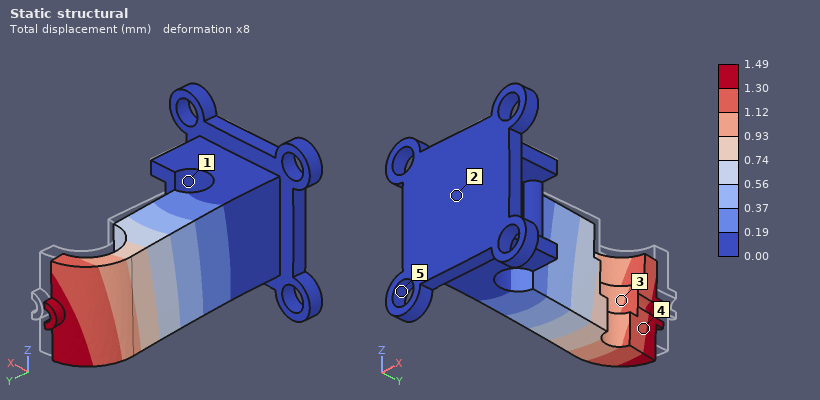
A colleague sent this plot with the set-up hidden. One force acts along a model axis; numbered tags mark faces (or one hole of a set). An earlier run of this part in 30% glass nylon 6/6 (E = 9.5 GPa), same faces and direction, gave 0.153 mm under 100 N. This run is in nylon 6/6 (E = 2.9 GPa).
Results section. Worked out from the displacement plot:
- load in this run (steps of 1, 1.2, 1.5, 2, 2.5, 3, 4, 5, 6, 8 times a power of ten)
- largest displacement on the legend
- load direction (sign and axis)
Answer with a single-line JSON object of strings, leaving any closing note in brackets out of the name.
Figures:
{"load in this run": "300 N", "largest displacement on the legend": "1.49 mm", "load direction": "-X"}
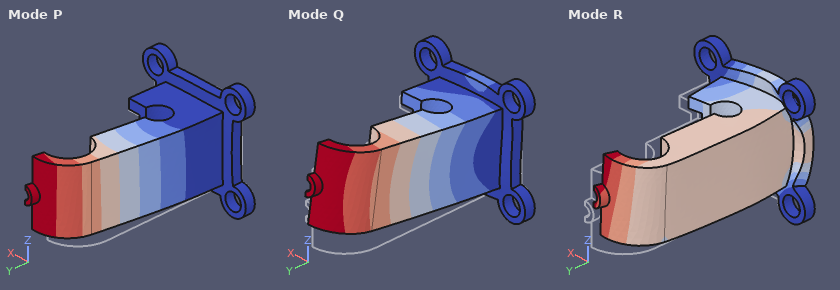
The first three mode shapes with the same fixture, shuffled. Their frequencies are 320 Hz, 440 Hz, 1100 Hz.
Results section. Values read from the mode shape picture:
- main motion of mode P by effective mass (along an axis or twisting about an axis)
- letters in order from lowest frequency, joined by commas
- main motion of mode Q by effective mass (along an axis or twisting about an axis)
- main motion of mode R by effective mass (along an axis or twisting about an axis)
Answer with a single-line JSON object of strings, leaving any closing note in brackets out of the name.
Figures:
{"main motion of mode P by effective mass": "along X", "letters in order from lowest frequency, joined by commas": "P, Q, R", "main motion of mode Q by effective mass": "along Z", "main motion of mode R by effective mass": "along Y"}
